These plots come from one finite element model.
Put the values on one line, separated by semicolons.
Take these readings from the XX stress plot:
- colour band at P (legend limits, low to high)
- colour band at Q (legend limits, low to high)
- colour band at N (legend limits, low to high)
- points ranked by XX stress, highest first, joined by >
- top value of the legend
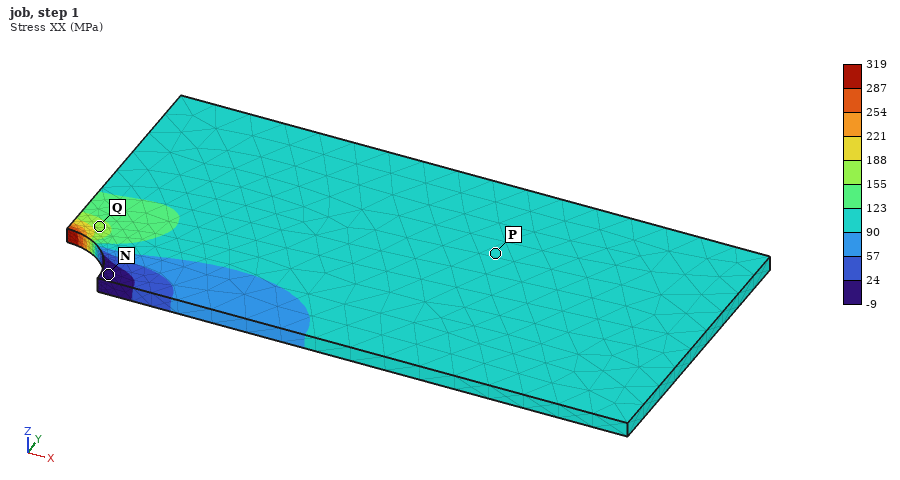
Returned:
90 to 123 MPa; 155 to 188 MPa; -9 to 24 MPa; Q > P > N; 319 MPa
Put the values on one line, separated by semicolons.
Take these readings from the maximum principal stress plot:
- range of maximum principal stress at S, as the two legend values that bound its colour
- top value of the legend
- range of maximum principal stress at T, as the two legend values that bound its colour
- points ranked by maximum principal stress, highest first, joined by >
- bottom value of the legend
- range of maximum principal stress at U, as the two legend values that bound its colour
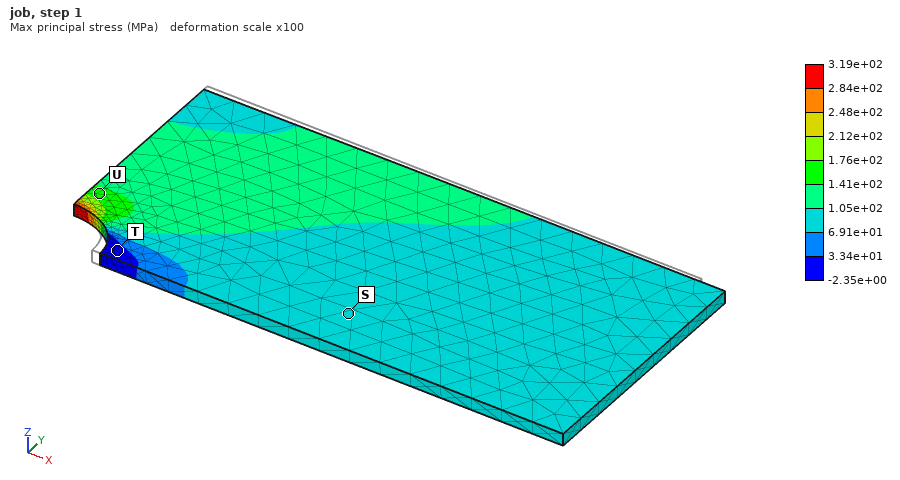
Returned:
6.91e+01 to 1.05e+02 MPa; 3.19e+02 MPa; -2.35e+00 to 3.34e+01 MPa; U > S > T; -2.35e+00 MPa; 1.41e+02 to 1.76e+02 MPa
